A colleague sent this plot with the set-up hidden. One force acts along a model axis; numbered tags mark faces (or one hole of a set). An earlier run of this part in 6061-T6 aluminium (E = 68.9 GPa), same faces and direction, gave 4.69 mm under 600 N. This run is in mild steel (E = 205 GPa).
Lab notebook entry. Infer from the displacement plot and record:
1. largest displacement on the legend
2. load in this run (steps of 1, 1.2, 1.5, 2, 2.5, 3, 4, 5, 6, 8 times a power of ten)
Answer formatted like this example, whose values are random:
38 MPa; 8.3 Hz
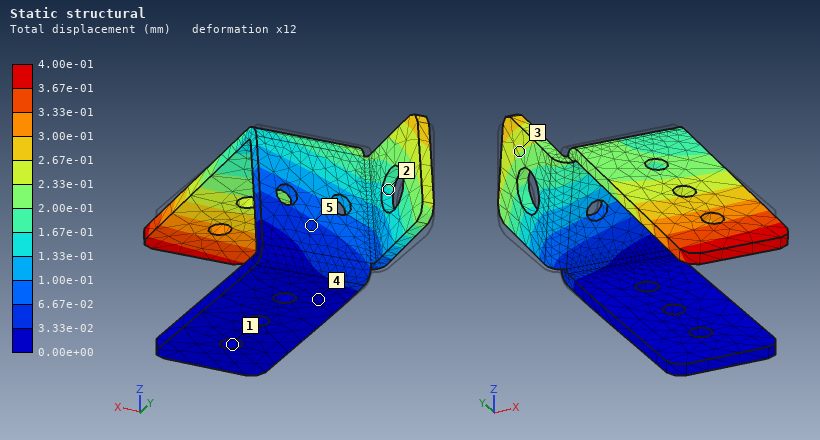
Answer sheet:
4.00e-01 mm; 150 N
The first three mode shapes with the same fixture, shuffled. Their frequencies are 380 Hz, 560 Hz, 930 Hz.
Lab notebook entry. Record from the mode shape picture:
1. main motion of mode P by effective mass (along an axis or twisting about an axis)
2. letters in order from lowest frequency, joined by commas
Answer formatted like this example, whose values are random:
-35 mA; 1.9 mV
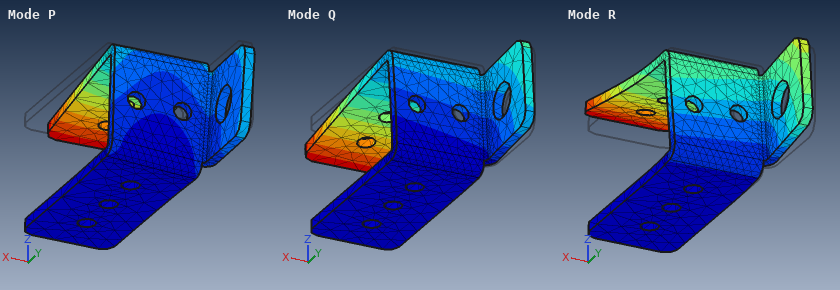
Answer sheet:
along X; Q, P, R
